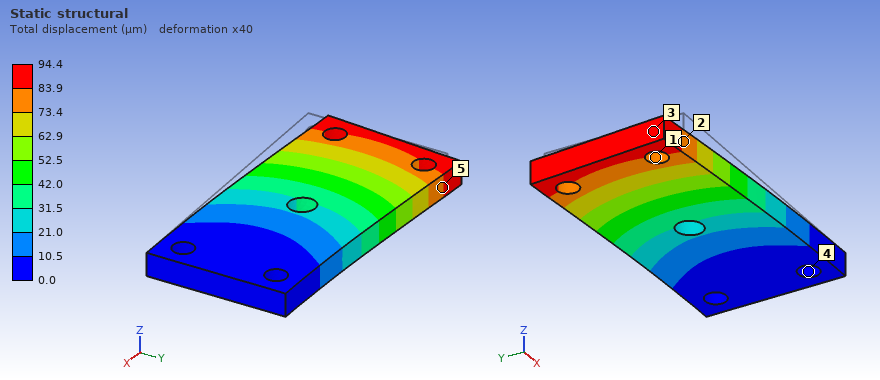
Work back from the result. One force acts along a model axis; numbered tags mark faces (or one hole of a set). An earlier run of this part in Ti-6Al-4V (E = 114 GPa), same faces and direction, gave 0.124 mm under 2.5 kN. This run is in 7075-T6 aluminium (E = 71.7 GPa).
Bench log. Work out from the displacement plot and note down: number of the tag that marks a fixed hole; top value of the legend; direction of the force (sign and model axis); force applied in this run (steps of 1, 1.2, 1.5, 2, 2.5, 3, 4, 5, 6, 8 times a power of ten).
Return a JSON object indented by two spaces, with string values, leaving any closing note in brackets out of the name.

{
  "number of the tag that marks a fixed hole": "4",
  "top value of the legend": "94.4 µm",
  "direction of the force": "+Y",
  "force applied in this run": "1.2 kN"
}
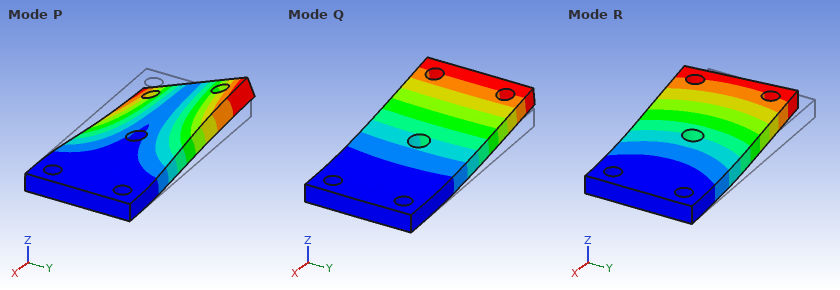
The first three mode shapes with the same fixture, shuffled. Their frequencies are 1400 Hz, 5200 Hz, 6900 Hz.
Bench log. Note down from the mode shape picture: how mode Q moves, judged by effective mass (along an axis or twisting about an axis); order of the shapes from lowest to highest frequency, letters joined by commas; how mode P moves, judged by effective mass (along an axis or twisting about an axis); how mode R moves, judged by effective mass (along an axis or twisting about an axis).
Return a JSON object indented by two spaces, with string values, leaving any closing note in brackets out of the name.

{
  "how mode Q moves, judged by effective mass": "along Z",
  "order of the shapes from lowest to highest frequency, letters joined by commas": "Q, P, R",
  "how mode P moves, judged by effective mass": "twisting about X",
  "how mode R moves, judged by effective mass": "along Y"
}
